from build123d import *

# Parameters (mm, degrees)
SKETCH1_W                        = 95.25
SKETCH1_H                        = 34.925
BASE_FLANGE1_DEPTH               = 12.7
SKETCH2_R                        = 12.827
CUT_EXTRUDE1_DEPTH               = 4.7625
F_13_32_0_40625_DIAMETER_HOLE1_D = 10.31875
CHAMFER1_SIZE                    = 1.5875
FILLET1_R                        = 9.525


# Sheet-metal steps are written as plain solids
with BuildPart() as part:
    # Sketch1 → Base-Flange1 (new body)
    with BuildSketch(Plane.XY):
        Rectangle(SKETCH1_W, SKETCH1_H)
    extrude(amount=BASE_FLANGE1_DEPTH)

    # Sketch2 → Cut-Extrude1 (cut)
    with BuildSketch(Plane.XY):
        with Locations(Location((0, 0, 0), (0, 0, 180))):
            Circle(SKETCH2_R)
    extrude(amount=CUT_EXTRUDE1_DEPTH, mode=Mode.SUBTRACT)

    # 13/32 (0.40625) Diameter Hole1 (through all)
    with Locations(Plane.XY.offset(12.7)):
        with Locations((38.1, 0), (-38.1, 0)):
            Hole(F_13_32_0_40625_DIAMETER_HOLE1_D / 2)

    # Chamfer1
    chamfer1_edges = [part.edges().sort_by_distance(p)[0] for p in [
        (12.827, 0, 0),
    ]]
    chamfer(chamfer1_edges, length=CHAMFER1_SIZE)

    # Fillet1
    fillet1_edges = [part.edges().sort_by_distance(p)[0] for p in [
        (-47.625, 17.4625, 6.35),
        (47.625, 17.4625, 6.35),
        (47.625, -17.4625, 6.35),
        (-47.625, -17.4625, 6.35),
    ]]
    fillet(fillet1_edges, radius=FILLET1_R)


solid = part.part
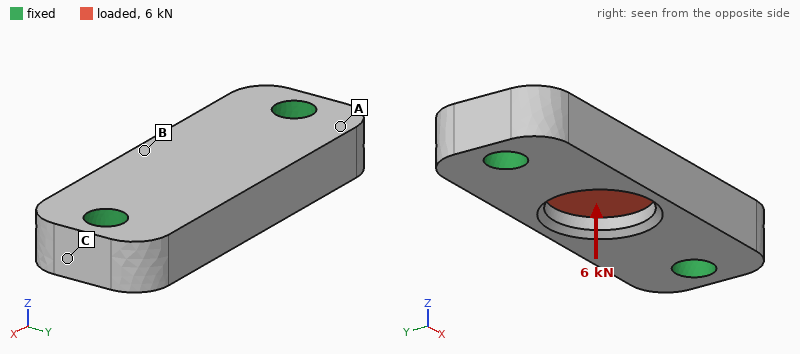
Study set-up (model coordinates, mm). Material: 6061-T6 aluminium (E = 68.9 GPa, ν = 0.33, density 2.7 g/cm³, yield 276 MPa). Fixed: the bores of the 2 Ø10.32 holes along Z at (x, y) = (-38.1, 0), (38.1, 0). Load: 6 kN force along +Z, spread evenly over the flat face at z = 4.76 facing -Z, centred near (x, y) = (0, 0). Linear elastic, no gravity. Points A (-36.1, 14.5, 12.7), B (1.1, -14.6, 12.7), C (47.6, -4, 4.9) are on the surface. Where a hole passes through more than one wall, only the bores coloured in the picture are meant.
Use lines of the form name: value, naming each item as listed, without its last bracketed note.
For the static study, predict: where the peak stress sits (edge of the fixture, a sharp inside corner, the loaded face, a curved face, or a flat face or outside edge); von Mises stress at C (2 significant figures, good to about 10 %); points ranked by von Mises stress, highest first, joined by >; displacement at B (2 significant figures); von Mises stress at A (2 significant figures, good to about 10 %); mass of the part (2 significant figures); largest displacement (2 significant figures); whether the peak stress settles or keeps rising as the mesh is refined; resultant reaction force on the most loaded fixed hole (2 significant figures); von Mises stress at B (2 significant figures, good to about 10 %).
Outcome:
where the peak stress sits: edge of the fixture
von Mises stress at C: 12 MPa
points ranked by von Mises stress, highest first, joined by >: B > A > C
displacement at B: 44 µm
von Mises stress at A: 20 MPa
mass of the part: 99 g
largest displacement: 49 µm
whether the peak stress settles or keeps rising as the mesh is refined: keeps rising
resultant reaction force on the most loaded fixed hole: 3.3 kN
von Mises stress at B: 55 MPa
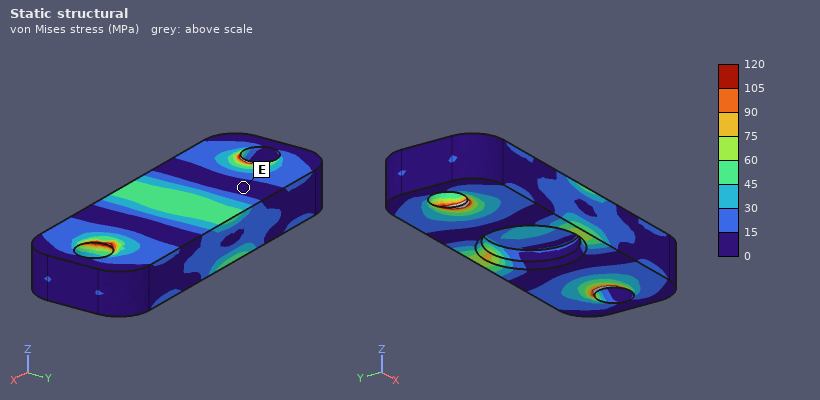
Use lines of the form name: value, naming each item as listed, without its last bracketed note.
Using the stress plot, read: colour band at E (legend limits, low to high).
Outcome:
colour band at E: 0 to 15 MPa
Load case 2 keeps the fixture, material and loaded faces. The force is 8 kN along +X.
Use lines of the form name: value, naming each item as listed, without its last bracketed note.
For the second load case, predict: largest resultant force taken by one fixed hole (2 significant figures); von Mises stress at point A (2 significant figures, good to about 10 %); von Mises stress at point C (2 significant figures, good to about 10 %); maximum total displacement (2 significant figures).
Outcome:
largest resultant force taken by one fixed hole: 4.0 kN
von Mises stress at point A: 4.6 MPa
von Mises stress at point C: 6.7 MPa
maximum total displacement: 9.7 µm
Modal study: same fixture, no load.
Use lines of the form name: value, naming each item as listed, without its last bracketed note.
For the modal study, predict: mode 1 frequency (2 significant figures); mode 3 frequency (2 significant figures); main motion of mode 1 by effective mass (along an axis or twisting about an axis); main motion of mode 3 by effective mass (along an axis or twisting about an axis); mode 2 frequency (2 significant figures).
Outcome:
mode 1 frequency: 10 kHz
mode 3 frequency: 15 kHz
main motion of mode 1 by effective mass: along Z
main motion of mode 3 by effective mass: along Y
mode 2 frequency: 13 kHz
